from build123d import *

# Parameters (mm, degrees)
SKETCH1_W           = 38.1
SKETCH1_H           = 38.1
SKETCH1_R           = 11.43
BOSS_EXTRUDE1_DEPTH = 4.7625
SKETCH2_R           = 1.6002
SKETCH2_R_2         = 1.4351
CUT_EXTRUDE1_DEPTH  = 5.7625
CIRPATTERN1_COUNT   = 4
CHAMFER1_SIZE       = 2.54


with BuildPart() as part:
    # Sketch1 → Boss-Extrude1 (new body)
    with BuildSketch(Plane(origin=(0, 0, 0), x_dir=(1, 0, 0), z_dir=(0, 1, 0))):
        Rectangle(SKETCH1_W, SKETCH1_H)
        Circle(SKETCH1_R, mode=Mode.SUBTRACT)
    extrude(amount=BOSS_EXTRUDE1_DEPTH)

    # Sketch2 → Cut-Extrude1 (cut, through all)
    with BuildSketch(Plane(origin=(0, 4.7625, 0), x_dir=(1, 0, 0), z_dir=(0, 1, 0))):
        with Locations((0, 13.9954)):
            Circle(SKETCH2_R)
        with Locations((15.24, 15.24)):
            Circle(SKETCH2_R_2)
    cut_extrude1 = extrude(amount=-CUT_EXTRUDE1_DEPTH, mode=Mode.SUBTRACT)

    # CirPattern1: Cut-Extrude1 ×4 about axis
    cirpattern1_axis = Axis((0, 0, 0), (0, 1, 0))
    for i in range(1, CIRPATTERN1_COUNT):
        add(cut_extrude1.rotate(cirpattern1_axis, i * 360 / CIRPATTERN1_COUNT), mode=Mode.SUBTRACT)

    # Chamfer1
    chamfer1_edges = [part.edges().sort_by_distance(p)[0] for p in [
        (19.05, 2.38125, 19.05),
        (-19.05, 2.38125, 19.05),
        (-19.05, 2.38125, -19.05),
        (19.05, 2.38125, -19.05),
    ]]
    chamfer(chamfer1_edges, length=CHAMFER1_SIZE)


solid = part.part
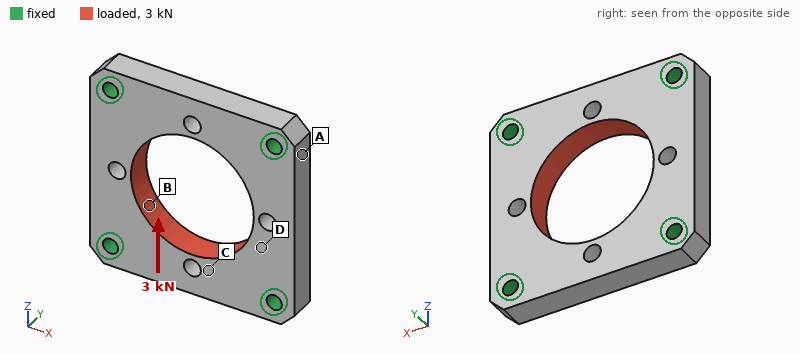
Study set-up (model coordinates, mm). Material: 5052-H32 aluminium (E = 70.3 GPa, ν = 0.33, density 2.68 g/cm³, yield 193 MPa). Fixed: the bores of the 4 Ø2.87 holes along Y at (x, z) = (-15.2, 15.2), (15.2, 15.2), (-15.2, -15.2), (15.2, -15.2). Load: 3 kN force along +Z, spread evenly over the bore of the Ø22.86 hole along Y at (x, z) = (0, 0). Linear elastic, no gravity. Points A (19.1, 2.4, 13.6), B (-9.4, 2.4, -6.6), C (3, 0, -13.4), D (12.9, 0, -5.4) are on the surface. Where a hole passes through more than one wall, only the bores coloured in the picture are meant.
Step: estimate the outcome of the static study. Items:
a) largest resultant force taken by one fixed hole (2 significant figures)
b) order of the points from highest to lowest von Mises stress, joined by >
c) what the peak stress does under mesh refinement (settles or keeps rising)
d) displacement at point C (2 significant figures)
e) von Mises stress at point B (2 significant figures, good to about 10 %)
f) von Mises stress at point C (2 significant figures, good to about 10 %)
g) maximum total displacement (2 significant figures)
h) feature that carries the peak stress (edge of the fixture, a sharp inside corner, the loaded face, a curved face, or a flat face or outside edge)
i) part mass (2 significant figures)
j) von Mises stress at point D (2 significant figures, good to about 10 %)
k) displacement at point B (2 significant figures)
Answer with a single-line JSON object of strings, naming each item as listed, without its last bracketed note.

{"largest resultant force taken by one fixed hole": "770 N", "order of the points from highest to lowest von Mises stress, joined by >": "B > D > C > A", "what the peak stress does under mesh refinement": "keeps rising", "displacement at point C": "7.6 µm", "von Mises stress at point B": "26 MPa", "von Mises stress at point C": "12 MPa", "maximum total displacement": "9.1 µm", "feature that carries the peak stress": "edge of the fixture", "part mass": "12 g", "von Mises stress at point D": "19 MPa", "displacement at point B": "4.4 µm"}
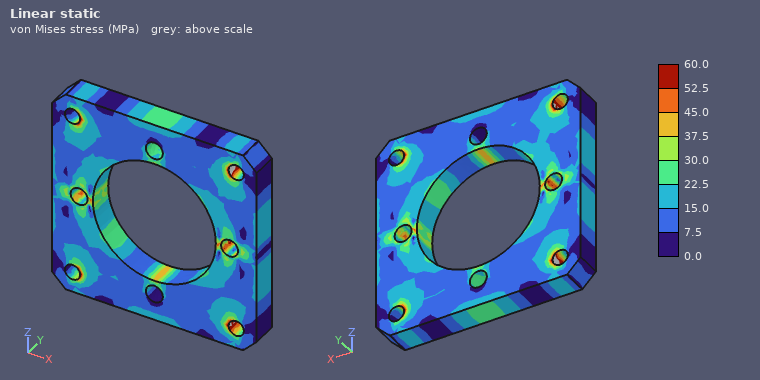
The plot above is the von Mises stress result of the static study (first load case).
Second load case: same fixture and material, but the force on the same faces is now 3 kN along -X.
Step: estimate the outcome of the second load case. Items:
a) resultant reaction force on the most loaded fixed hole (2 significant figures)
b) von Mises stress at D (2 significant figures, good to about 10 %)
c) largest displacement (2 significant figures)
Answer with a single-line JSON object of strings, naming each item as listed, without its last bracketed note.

{"resultant reaction force on the most loaded fixed hole": "770 N", "von Mises stress at D": "14 MPa", "largest displacement": "9.1 µm"}
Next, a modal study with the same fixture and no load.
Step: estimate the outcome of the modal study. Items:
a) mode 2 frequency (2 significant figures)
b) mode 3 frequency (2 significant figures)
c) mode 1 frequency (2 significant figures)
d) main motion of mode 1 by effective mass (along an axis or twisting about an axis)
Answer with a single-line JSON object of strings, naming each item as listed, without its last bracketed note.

{"mode 2 frequency": "25 kHz", "mode 3 frequency": "25 kHz", "mode 1 frequency": "23 kHz", "main motion of mode 1 by effective mass": "along Y"}
